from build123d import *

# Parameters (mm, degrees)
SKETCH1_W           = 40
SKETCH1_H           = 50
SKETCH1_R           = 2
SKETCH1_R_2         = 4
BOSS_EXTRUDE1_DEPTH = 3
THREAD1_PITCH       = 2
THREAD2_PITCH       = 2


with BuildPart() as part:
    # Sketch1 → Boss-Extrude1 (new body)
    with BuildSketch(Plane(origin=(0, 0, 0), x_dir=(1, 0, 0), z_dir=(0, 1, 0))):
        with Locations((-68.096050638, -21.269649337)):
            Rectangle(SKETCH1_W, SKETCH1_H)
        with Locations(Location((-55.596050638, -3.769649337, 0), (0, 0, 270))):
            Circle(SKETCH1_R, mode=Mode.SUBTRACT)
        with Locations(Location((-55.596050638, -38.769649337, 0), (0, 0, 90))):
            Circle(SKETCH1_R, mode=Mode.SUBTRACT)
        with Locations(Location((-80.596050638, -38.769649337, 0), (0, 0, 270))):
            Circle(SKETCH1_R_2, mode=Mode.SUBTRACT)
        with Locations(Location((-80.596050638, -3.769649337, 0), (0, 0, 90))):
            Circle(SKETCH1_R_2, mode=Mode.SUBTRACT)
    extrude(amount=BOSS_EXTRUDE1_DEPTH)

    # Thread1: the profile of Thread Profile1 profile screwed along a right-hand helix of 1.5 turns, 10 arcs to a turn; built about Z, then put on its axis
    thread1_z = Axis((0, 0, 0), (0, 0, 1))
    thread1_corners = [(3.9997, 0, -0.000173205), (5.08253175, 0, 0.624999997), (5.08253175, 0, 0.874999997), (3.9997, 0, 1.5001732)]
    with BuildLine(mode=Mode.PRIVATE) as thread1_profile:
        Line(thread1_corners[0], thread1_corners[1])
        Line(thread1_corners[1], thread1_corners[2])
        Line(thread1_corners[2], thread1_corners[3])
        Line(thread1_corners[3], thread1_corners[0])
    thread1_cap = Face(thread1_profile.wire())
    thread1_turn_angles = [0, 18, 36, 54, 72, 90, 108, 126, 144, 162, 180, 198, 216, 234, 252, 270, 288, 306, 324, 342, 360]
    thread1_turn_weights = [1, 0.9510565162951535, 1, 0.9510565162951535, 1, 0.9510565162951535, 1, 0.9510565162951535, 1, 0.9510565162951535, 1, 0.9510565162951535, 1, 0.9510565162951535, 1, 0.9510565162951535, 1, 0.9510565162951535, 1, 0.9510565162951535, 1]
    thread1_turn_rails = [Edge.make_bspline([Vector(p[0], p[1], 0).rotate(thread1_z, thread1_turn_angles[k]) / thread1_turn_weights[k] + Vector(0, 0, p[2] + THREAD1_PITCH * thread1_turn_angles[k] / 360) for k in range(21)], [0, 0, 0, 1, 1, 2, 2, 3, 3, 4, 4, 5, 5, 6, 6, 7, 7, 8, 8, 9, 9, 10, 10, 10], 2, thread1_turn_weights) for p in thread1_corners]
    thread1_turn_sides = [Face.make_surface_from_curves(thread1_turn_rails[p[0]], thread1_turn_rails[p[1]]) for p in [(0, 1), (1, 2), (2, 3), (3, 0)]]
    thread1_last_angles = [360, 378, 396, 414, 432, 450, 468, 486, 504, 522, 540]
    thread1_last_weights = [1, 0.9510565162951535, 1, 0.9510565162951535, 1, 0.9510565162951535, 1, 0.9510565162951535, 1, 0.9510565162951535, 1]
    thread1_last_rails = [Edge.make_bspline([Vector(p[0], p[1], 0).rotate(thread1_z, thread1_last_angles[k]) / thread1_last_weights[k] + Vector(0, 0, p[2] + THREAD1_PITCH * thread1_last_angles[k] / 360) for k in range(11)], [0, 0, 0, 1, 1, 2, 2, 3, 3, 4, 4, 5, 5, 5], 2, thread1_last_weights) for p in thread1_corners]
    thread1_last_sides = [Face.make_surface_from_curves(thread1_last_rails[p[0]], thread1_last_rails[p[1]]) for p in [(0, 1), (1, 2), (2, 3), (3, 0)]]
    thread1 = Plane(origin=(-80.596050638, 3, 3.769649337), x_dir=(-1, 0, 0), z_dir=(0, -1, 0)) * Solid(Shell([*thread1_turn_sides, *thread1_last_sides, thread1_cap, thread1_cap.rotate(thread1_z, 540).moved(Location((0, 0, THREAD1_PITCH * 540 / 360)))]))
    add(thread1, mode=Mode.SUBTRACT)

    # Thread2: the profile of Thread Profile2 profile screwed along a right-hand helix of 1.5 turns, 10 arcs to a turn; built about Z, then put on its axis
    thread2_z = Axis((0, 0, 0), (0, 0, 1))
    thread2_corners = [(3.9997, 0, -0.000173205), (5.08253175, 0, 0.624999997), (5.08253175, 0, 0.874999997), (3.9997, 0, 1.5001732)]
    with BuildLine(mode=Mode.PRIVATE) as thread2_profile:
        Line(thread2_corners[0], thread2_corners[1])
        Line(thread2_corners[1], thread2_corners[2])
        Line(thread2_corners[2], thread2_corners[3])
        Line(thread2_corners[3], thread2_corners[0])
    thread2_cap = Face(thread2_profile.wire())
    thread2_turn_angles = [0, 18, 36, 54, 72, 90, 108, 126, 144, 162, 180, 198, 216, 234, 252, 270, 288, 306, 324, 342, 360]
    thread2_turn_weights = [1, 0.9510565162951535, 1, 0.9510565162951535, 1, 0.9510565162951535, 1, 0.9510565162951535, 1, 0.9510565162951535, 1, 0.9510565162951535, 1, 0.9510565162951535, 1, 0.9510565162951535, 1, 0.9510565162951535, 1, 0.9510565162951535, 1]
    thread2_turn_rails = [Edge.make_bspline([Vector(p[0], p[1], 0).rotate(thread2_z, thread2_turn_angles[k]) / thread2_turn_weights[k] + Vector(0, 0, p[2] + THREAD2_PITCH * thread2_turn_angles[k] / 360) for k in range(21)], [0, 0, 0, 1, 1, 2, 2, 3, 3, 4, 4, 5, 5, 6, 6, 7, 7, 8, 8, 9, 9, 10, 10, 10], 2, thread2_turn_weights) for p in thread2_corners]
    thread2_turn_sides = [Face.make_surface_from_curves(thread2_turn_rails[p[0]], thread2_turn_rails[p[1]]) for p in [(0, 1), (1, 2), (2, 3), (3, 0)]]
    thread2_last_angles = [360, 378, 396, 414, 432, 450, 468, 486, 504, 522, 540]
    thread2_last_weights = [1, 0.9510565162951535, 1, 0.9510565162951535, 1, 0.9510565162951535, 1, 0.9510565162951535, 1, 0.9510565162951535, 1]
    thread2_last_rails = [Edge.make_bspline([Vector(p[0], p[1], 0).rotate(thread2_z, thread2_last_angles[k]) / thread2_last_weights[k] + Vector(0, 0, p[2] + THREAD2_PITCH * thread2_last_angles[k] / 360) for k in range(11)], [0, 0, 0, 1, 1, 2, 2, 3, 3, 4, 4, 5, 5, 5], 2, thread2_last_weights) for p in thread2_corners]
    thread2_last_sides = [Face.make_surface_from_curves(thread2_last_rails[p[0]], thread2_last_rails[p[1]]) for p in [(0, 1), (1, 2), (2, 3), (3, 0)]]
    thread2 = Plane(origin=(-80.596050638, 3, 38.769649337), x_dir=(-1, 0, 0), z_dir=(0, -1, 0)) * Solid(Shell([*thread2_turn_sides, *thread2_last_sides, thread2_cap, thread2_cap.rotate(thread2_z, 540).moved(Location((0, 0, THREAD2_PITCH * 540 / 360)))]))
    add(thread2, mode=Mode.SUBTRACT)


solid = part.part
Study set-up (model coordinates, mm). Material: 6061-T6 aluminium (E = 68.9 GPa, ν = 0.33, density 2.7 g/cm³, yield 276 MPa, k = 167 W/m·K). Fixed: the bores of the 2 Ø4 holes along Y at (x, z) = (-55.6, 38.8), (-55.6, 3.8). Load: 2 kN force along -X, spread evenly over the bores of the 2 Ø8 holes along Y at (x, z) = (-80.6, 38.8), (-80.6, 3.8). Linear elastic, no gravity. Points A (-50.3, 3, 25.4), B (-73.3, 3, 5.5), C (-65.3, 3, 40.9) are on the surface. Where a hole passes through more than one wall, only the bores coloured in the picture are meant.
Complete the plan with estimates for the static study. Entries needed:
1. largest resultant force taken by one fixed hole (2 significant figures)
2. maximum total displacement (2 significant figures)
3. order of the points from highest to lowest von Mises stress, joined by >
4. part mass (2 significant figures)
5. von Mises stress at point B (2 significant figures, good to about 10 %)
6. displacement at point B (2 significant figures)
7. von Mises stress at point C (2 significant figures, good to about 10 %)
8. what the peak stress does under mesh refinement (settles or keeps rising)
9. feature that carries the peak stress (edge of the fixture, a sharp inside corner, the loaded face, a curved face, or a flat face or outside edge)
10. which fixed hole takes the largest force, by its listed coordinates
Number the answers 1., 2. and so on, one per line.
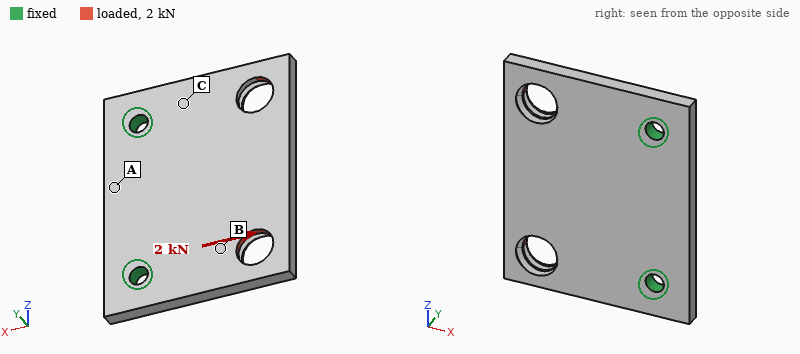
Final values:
1. 1.1 kN
2. 72 µm
3. B > C > A
4. 15 g
5. 39 MPa
6. 24 µm
7. 24 MPa
8. keeps rising
9. a sharp inside corner
10. (-55.6, 3.8)
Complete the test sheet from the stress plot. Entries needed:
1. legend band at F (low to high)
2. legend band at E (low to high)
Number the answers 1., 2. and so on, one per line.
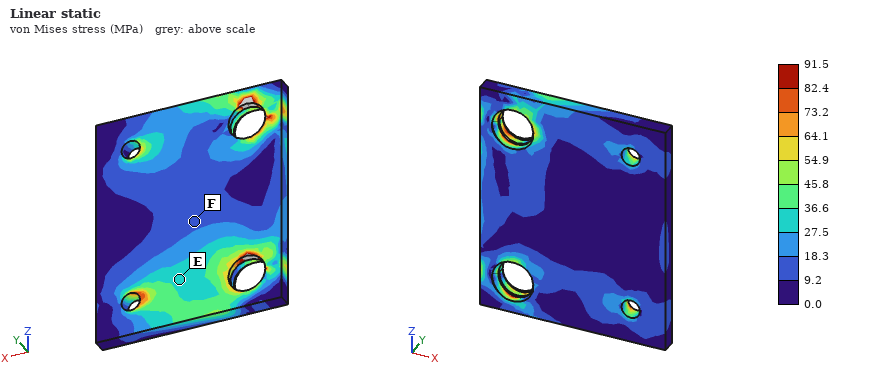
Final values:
1. 9.2 to 18.3 MPa
2. 27.5 to 36.6 MPa
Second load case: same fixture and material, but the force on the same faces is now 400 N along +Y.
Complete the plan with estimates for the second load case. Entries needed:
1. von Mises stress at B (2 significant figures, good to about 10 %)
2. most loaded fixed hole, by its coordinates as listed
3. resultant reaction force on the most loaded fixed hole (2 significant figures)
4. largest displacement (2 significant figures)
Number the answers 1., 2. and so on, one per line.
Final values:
1. 40 MPa
2. (-55.6, 3.8)
3. 220 N
4. 0.47 mm
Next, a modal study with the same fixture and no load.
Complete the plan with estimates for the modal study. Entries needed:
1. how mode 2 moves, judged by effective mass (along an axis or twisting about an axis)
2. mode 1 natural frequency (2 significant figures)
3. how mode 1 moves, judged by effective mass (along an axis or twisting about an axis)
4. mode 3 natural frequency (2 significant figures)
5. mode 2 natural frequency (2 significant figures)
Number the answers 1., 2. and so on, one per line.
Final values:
1. twisting about X
2. 2300 Hz
3. along Y
4. 8700 Hz
5. 4600 Hz
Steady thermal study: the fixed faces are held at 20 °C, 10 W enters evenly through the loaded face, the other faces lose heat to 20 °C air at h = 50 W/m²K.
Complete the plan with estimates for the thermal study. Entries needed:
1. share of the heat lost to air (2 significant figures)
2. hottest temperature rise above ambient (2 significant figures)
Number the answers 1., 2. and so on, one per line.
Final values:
1. 14 %
2. 16 K
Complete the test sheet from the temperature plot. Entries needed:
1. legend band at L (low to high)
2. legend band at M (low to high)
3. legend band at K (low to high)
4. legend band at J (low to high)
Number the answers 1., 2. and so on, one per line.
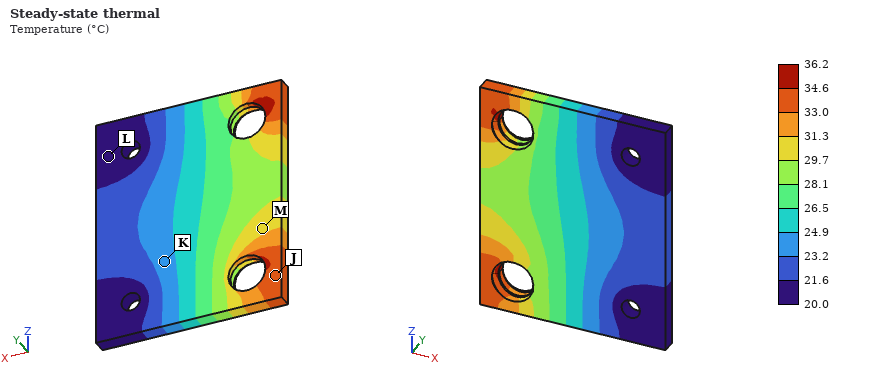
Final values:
1. 20.0 to 21.6 °C
2. 29.7 to 31.3 °C
3. 23.2 to 24.9 °C
4. 33.0 to 34.6 °C
